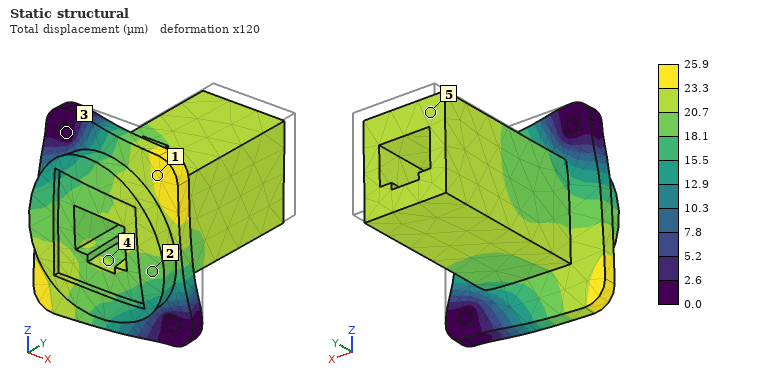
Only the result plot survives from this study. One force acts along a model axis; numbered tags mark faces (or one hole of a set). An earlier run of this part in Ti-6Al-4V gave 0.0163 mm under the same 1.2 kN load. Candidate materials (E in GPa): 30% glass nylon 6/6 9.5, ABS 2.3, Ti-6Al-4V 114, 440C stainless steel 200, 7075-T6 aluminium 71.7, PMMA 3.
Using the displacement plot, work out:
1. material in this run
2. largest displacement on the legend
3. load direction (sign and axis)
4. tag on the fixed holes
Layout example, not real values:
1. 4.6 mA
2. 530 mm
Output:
1. 7075-T6 aluminium
2. 25.9 µm
3. -Y
4. 3
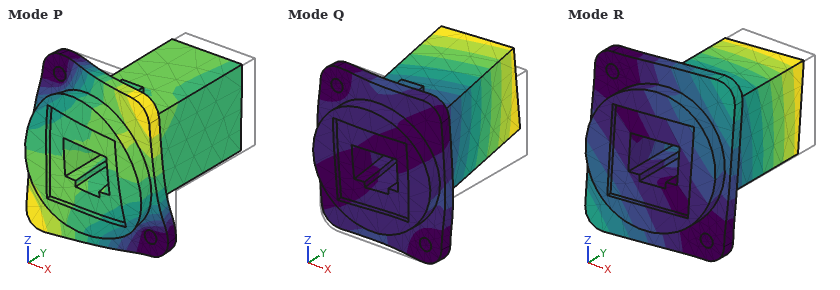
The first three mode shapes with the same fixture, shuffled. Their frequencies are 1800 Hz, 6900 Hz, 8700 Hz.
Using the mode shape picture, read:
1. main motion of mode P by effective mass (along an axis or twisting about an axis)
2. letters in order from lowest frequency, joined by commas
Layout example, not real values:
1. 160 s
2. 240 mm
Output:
1. along Y
2. R, Q, P
